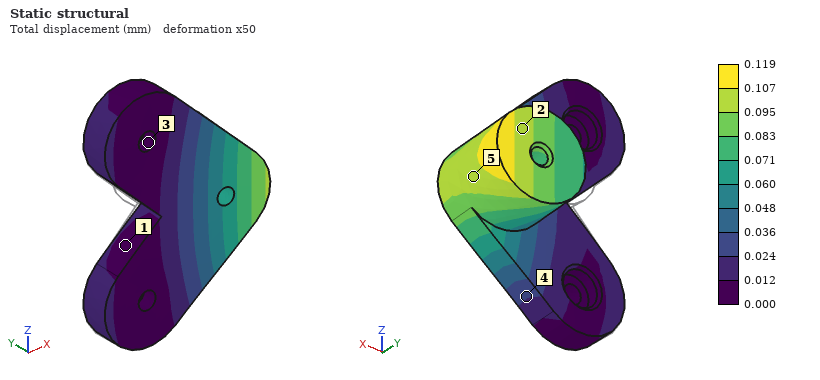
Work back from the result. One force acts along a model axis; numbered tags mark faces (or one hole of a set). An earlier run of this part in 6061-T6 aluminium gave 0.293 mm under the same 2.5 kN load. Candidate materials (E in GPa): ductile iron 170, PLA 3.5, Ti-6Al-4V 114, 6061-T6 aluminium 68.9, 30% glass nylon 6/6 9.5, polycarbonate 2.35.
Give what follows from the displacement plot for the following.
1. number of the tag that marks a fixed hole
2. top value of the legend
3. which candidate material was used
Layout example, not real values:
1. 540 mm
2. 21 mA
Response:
1. 3
2. 0.119 mm
3. ductile iron
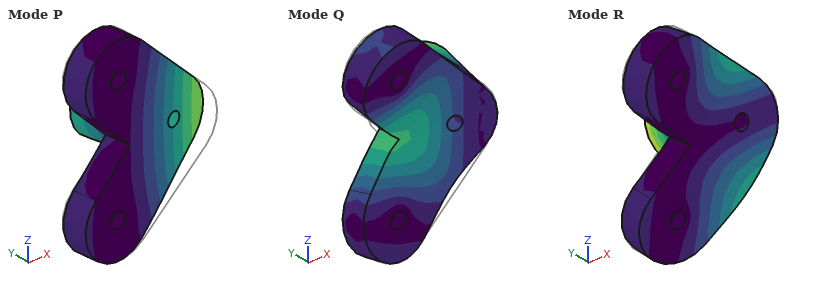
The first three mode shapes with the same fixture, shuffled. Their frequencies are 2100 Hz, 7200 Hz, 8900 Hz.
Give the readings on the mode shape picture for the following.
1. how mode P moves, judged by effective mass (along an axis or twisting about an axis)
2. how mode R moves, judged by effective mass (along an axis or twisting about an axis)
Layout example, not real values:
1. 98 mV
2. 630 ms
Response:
1. along Y
2. along Z
